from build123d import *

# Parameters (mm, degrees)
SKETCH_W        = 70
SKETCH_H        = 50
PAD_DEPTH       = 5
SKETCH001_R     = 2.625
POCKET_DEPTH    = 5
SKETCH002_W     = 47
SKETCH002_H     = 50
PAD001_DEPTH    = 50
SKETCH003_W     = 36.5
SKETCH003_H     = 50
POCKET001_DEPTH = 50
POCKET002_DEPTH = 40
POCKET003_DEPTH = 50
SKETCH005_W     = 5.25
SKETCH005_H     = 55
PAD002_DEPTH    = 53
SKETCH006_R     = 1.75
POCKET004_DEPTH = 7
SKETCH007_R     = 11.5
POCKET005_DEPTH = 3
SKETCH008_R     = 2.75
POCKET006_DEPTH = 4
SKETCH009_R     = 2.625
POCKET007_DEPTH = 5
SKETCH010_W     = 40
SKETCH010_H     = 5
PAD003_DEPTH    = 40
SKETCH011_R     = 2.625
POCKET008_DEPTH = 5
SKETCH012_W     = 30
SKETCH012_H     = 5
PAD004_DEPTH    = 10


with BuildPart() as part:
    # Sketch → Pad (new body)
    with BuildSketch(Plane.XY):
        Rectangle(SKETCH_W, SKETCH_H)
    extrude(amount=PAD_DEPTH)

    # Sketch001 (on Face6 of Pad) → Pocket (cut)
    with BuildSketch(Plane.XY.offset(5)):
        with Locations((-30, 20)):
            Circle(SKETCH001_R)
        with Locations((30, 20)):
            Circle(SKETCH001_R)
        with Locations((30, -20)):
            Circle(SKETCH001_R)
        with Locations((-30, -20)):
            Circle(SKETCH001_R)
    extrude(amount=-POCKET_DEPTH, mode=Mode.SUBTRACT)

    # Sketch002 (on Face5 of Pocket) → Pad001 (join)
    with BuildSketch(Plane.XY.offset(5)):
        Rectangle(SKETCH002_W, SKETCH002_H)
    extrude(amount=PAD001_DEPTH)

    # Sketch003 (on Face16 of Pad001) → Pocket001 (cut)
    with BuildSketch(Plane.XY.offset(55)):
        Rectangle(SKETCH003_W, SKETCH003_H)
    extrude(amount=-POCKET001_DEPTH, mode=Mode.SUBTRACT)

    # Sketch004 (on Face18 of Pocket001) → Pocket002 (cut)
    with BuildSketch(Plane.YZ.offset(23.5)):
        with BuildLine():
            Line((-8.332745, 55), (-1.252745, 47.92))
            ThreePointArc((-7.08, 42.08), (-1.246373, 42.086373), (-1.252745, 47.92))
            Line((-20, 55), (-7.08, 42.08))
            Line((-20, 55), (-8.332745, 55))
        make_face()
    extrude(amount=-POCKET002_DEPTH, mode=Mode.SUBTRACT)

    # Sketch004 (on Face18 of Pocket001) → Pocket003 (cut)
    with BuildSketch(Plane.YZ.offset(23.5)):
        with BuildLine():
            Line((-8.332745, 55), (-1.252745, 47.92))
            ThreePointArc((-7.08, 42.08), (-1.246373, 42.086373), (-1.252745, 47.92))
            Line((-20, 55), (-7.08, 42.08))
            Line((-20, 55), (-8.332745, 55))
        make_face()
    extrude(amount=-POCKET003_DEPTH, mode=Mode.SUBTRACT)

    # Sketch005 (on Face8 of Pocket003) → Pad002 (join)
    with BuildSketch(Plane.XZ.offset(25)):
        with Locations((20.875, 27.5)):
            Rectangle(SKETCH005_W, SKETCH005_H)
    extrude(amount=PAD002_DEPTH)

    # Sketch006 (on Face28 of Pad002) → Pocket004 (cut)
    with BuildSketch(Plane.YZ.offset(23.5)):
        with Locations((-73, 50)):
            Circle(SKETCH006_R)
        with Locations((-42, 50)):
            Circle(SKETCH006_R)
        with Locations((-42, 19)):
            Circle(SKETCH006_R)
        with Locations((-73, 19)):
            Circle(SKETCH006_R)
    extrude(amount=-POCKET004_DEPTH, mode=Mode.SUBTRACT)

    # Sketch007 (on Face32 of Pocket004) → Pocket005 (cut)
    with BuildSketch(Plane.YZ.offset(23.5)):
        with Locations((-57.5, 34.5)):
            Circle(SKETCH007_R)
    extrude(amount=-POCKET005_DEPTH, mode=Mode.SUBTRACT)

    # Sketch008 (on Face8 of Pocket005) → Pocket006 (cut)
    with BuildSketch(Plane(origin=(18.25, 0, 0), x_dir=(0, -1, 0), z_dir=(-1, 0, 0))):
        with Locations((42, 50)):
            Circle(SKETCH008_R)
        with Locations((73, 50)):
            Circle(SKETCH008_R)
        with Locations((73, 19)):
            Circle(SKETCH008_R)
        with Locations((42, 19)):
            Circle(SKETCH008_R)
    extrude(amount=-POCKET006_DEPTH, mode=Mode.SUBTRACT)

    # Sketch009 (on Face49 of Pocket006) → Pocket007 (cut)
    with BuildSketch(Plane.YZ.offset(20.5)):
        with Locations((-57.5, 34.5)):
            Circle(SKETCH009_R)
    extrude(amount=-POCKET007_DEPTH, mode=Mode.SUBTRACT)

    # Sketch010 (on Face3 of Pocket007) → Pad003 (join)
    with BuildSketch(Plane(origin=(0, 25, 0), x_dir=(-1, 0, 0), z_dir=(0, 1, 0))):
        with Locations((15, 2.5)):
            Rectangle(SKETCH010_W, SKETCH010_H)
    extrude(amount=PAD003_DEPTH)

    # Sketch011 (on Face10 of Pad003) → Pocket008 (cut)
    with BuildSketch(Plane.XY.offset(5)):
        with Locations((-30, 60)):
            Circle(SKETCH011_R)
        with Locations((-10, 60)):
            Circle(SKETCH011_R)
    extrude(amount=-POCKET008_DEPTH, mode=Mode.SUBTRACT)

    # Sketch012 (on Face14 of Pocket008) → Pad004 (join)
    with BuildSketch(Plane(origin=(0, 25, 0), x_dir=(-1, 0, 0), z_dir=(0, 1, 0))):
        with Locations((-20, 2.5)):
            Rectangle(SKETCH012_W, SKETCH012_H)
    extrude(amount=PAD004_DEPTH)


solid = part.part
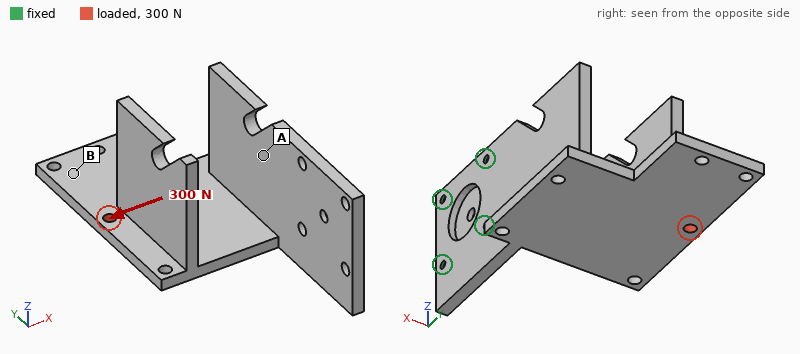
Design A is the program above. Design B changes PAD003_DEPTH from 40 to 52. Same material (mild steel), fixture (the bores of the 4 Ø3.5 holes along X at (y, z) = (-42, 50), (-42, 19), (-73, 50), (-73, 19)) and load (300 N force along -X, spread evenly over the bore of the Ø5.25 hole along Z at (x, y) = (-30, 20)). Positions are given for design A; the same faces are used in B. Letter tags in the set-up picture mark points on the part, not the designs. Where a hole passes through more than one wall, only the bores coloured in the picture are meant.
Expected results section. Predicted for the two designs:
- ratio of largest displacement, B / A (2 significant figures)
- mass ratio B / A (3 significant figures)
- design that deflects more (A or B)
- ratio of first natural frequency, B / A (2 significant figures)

1.1
1.04
B
0.92
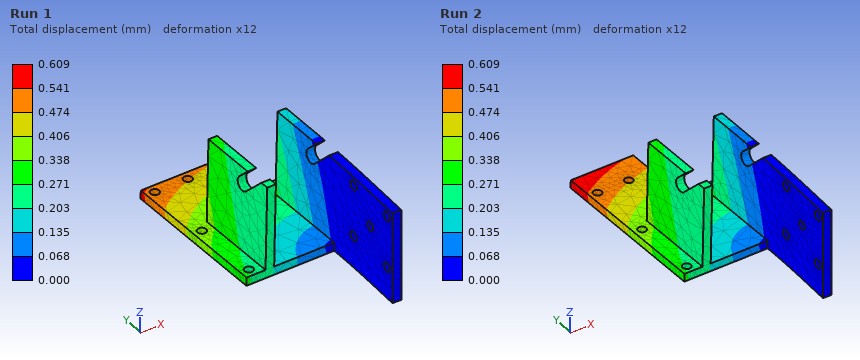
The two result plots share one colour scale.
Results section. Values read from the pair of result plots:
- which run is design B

Run 2
